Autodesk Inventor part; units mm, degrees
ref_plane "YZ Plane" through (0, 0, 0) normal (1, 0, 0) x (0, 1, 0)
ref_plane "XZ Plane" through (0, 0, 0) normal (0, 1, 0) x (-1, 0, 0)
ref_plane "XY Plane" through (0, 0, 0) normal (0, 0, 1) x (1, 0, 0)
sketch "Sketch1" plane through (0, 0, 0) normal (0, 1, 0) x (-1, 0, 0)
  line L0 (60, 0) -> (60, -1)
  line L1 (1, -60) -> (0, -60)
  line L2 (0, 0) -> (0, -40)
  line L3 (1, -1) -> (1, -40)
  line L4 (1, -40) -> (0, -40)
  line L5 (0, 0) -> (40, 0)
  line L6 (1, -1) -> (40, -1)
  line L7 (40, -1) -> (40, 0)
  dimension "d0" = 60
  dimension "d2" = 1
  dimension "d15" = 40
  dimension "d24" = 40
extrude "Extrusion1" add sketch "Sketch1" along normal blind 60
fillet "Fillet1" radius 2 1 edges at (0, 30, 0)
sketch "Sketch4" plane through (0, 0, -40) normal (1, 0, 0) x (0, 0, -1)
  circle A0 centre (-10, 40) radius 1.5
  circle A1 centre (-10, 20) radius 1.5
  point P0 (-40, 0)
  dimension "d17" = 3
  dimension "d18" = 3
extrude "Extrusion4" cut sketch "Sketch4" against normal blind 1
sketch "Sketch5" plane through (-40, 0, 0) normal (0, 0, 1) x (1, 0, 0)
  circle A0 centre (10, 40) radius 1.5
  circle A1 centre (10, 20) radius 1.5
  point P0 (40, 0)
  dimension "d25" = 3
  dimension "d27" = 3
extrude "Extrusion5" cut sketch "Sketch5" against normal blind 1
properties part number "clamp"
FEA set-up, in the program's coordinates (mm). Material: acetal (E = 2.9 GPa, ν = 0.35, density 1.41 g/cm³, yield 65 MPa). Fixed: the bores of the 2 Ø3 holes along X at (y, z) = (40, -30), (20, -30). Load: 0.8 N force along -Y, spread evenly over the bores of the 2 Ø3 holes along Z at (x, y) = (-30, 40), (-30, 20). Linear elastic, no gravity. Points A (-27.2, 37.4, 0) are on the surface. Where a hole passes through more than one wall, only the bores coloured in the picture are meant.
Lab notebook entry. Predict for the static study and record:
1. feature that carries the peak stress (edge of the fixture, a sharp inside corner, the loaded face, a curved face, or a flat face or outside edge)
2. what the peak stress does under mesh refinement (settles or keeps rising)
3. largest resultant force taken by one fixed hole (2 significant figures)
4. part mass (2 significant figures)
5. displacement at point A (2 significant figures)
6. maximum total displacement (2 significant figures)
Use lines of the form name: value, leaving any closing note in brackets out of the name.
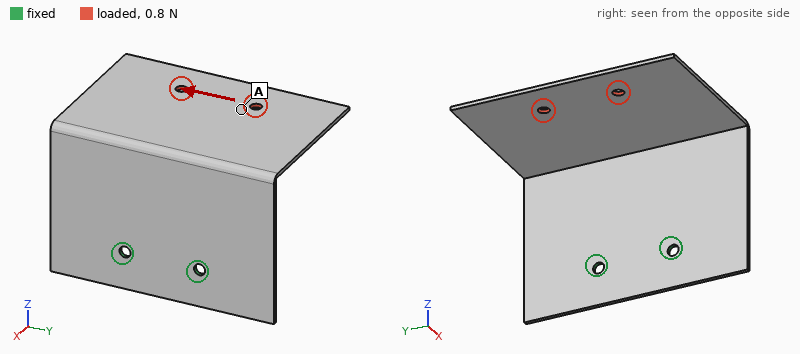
feature that carries the peak stress: edge of the fixture
what the peak stress does under mesh refinement: keeps rising
largest resultant force taken by one fixed hole: 1.4 N
part mass: 6.6 g
displacement at point A: 0.52 mm
maximum total displacement: 0.96 mm
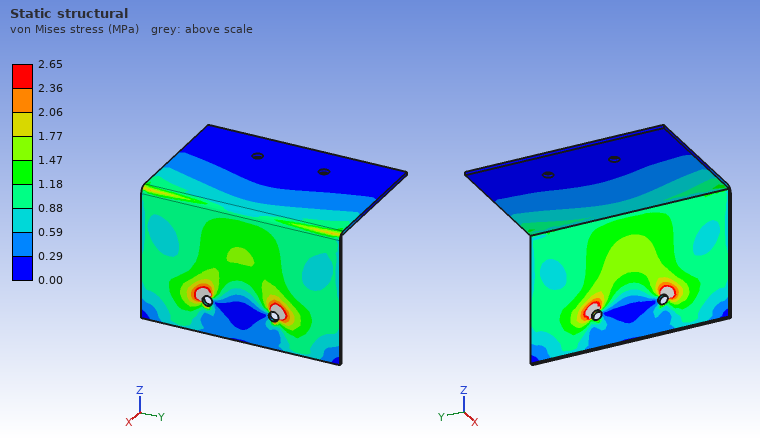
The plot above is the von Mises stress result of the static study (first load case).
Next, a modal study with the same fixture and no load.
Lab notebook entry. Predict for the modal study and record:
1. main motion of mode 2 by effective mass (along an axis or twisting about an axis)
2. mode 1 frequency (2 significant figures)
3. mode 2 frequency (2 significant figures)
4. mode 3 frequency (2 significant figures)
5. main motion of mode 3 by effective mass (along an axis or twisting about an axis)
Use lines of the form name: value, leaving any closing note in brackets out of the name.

main motion of mode 2 by effective mass: along Y
mode 1 frequency: 64 Hz
mode 2 frequency: 100 Hz
mode 3 frequency: 170 Hz
main motion of mode 3 by effective mass: along X
